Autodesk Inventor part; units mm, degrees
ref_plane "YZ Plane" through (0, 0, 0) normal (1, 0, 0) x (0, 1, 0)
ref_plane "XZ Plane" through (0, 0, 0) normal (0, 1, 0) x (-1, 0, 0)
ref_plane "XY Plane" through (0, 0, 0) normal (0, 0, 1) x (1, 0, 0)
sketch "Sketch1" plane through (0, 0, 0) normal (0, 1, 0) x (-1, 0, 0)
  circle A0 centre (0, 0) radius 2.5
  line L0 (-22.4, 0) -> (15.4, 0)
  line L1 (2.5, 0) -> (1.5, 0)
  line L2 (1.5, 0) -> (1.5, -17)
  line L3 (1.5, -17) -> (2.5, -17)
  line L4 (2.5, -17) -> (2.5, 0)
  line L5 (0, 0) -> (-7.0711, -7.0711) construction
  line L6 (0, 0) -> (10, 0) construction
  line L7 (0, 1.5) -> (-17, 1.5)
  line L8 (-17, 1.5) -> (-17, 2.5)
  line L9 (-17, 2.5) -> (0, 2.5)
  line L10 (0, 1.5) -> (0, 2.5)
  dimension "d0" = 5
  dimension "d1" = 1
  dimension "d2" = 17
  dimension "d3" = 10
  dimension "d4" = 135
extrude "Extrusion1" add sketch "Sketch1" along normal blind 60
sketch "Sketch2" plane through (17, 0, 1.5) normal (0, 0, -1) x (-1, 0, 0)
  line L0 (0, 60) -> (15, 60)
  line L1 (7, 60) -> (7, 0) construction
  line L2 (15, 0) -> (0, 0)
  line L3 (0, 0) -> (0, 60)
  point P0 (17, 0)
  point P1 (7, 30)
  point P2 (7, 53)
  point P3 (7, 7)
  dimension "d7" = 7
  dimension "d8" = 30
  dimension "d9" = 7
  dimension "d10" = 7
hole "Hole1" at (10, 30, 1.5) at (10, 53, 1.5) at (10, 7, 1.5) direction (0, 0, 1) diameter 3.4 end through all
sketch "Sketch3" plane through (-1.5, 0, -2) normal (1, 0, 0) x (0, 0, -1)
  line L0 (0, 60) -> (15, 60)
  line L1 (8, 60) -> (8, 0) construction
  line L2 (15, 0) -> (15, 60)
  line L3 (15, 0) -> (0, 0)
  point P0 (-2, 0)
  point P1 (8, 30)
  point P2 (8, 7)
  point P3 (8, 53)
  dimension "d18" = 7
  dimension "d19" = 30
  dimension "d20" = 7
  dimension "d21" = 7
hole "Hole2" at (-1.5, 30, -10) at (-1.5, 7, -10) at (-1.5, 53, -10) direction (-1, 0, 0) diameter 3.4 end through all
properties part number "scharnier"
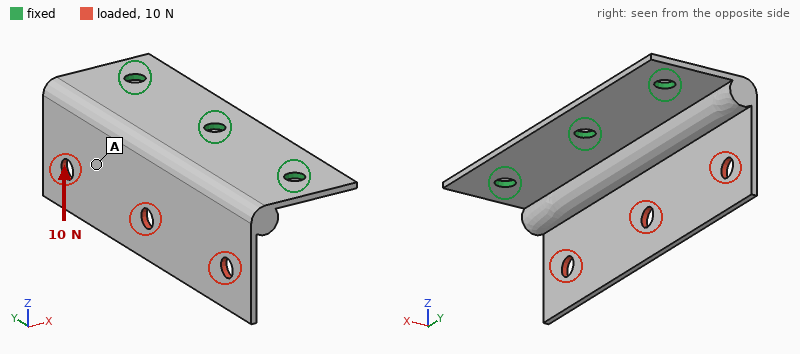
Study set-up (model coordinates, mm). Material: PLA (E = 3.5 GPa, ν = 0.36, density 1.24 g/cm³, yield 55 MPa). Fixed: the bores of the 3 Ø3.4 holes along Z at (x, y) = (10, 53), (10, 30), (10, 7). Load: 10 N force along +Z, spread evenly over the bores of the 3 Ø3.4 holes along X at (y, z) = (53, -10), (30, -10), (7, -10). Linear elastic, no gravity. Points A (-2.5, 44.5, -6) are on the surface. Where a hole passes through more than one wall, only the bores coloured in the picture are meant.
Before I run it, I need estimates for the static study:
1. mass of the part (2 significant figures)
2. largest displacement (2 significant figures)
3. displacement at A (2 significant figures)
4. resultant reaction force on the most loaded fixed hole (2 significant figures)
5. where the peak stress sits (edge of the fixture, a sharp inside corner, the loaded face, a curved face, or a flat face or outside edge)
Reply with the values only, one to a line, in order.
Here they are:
3.7 g
0.69 mm
0.40 mm
3.4 N
a flat face or outside edge
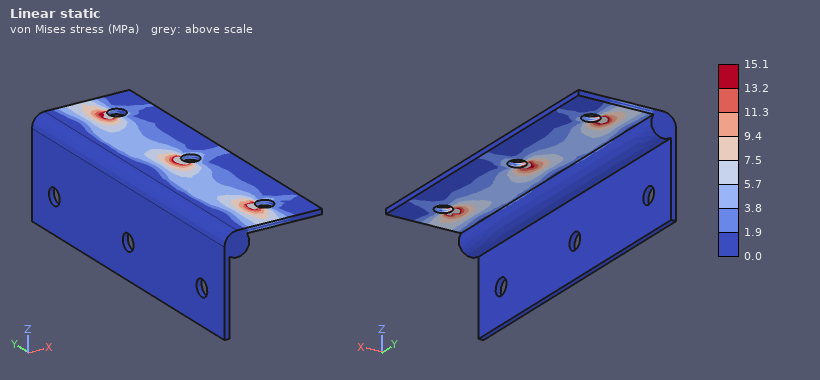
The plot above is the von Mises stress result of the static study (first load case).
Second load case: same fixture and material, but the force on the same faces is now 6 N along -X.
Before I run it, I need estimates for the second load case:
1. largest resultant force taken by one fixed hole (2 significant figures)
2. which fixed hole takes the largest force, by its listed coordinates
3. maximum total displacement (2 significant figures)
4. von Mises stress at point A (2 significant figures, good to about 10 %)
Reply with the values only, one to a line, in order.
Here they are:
2.6 N
(10, 30)
0.79 mm
2.2 MPa
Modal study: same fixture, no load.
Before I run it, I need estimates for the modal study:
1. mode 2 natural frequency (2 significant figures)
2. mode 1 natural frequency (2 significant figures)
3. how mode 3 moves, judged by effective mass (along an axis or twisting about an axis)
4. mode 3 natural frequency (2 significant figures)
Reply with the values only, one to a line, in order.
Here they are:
1000 Hz
430 Hz
along Z
1400 Hz
